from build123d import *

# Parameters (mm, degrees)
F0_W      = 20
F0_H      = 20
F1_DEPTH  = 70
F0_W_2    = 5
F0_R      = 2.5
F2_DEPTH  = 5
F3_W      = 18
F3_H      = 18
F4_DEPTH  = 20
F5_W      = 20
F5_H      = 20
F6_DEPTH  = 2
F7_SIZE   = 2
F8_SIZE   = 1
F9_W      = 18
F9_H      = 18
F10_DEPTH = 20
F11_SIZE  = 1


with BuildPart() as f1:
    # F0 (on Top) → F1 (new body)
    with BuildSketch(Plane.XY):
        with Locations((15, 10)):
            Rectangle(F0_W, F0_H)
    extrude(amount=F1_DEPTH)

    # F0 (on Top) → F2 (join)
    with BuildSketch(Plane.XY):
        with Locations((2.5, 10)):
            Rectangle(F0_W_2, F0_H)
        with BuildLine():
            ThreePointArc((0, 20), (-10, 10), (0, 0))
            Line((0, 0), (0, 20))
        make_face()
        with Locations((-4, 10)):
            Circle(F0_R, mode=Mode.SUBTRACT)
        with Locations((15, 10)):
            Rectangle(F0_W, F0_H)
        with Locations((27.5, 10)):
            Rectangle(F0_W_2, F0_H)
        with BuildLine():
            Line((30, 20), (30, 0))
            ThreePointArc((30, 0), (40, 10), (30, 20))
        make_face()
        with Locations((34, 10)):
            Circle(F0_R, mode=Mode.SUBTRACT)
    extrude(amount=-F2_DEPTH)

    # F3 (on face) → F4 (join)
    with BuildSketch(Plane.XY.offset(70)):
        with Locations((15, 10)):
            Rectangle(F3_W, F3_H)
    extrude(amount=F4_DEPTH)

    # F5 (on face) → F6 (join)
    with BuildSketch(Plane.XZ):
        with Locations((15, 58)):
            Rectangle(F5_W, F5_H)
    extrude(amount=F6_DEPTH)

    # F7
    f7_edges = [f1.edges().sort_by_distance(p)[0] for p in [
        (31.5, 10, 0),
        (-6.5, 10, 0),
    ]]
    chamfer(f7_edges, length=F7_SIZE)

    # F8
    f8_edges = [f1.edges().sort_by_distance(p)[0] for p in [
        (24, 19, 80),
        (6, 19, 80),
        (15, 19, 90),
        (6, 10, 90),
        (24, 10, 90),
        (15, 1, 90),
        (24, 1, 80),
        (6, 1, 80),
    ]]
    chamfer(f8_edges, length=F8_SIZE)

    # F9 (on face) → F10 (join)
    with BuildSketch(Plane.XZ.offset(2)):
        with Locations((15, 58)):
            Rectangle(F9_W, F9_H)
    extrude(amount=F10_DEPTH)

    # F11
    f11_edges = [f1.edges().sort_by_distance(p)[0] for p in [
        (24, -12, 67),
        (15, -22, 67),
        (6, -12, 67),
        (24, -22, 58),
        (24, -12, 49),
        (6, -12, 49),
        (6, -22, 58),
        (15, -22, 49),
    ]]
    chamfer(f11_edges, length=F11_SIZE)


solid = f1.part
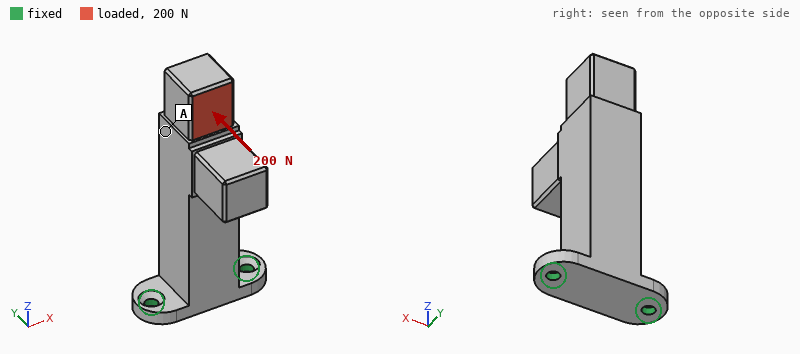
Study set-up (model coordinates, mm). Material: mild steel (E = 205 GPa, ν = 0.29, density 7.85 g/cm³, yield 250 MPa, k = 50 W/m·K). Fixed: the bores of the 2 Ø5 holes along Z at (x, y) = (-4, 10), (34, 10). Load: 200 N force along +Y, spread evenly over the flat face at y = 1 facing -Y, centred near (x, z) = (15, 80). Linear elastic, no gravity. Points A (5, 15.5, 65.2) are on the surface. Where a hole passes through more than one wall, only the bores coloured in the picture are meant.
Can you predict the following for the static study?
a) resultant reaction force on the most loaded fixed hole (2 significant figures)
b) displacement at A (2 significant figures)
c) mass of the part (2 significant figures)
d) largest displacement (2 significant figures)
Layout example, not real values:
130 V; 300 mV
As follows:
100 N; 0.12 mm; 360 g; 0.17 mm
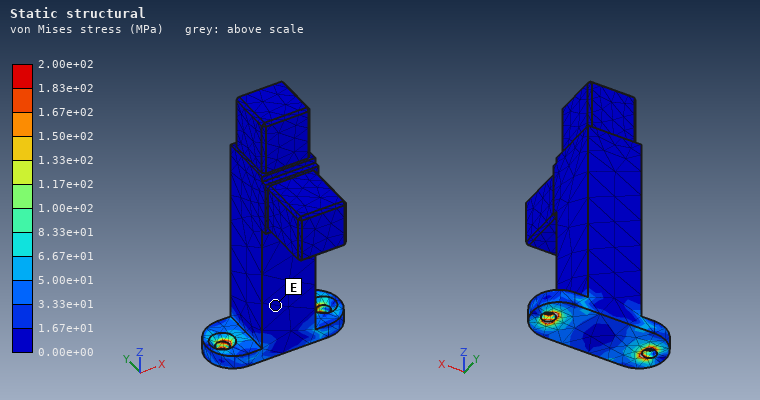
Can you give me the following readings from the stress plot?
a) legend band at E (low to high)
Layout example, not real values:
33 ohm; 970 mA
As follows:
0.00e+00 to 1.67e+01 MPa
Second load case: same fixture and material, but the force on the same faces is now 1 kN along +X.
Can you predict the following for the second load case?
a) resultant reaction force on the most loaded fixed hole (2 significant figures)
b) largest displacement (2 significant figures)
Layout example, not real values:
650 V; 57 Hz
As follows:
2.7 kN; 0.18 mm
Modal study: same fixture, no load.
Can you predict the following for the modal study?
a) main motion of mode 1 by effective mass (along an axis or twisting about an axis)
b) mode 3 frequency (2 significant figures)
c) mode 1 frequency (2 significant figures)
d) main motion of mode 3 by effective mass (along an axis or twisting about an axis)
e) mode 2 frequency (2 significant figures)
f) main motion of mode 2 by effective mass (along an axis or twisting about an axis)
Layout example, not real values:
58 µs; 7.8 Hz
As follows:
along Y; 4600 Hz; 490 Hz; twisting about Z; 1100 Hz; along X
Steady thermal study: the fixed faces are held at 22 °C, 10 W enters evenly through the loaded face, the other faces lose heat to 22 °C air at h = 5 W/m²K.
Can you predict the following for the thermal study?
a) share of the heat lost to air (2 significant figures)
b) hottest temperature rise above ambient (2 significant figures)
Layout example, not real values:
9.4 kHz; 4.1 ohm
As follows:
14 %; 51 K
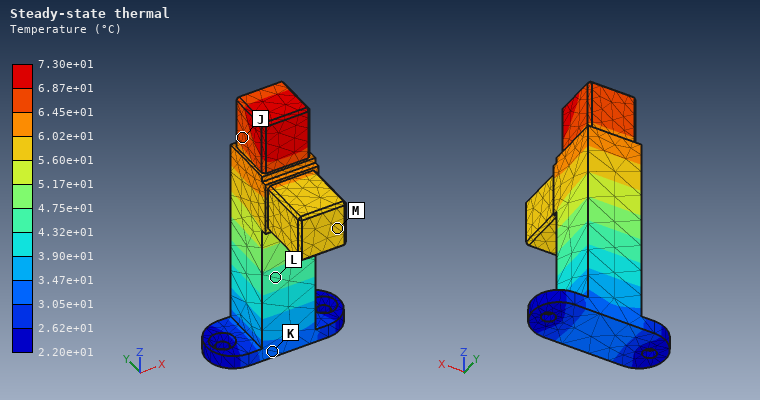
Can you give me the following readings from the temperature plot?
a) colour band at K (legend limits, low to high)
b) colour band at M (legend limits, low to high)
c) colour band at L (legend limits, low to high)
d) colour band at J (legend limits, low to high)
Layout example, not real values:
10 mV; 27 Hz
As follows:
3.05e+01 to 3.47e+01 °C; 5.60e+01 to 6.02e+01 °C; 4.32e+01 to 4.75e+01 °C; 6.45e+01 to 6.87e+01 °C
